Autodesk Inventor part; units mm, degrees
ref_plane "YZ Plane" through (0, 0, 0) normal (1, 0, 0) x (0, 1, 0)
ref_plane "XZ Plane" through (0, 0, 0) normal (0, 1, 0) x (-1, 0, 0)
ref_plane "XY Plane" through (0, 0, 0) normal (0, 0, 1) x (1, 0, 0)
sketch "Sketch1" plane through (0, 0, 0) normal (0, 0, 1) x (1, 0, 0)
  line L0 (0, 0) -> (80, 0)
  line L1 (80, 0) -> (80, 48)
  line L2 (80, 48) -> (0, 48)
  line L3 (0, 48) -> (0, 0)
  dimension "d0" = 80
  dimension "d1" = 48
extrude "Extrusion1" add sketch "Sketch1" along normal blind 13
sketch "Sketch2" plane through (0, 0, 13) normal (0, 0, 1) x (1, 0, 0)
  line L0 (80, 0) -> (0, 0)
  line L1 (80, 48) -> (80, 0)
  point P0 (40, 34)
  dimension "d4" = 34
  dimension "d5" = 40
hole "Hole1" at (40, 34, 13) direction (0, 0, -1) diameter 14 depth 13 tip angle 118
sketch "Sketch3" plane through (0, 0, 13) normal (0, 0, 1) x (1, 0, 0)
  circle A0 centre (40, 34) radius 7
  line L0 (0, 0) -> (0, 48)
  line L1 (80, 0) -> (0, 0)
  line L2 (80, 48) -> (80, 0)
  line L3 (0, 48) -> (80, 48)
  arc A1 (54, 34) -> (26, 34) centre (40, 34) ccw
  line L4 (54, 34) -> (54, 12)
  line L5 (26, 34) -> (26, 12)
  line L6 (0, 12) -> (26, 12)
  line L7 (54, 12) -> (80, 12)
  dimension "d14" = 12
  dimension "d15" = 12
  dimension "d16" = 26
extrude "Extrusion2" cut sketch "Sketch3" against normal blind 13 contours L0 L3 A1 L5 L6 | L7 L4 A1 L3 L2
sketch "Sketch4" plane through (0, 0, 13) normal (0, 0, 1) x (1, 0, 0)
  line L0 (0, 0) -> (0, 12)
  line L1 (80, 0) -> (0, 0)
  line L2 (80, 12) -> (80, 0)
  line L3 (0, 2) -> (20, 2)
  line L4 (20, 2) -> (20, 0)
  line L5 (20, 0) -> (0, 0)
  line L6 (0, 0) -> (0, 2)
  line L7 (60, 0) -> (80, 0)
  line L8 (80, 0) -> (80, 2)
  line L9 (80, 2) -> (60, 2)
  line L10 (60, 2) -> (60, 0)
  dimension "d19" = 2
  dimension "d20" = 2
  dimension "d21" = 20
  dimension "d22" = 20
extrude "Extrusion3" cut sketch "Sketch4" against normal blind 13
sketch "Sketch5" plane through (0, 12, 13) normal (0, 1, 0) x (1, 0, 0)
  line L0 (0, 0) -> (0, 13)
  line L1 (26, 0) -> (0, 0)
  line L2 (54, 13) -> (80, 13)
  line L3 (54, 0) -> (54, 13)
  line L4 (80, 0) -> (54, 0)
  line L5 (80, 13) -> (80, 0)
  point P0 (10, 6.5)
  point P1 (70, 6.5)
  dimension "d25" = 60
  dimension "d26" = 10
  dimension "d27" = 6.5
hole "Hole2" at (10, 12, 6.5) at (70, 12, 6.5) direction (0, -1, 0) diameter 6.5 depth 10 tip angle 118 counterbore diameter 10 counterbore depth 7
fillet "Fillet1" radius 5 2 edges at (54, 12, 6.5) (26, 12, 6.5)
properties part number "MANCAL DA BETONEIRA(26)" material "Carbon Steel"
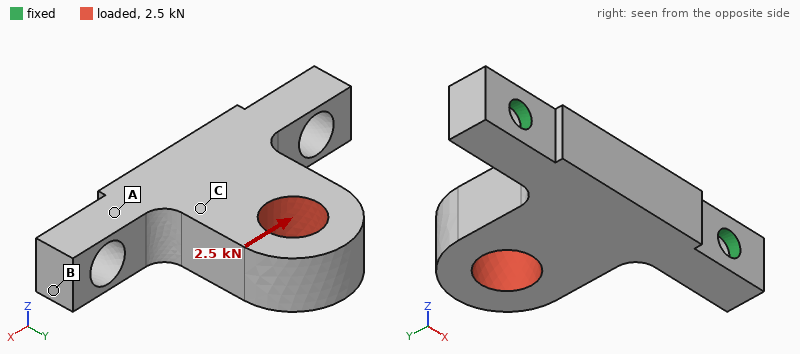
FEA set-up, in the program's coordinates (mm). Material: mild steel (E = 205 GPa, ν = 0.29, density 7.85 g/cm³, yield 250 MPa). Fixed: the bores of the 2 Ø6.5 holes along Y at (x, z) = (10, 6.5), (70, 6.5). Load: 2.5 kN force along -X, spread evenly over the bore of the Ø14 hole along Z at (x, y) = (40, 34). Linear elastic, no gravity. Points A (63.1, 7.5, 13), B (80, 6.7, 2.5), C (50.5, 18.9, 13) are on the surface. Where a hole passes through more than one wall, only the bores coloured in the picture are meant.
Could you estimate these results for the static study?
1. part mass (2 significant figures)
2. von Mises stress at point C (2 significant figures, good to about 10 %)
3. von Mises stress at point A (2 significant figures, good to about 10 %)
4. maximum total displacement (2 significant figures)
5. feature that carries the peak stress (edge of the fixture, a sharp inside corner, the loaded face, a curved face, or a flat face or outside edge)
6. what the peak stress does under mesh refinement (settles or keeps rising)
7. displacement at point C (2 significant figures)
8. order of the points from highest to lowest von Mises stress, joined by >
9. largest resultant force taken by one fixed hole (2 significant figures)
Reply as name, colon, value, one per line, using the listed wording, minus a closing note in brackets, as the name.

part mass: 160 g
von Mises stress at point C: 19 MPa
von Mises stress at point A: 33 MPa
maximum total displacement: 20 µm
feature that carries the peak stress: edge of the fixture
what the peak stress does under mesh refinement: keeps rising
displacement at point C: 5.3 µm
order of the points from highest to lowest von Mises stress, joined by >: A > C > B
largest resultant force taken by one fixed hole: 1.9 kN
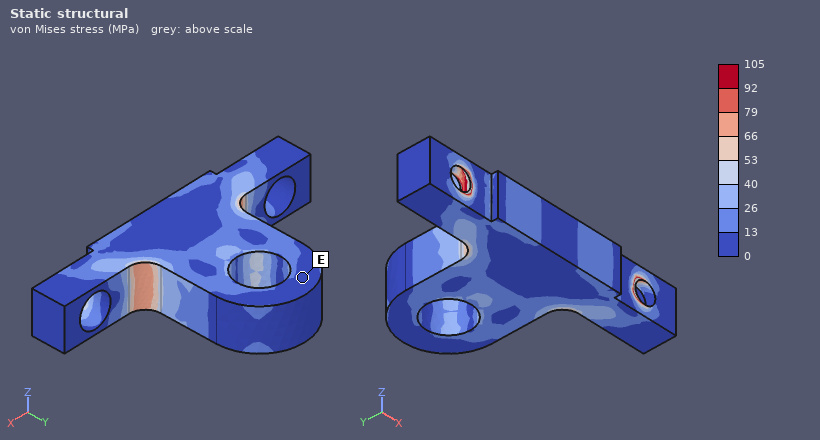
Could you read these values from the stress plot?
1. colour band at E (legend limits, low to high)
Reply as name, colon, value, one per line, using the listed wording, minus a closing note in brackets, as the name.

colour band at E: 0 to 13 MPa
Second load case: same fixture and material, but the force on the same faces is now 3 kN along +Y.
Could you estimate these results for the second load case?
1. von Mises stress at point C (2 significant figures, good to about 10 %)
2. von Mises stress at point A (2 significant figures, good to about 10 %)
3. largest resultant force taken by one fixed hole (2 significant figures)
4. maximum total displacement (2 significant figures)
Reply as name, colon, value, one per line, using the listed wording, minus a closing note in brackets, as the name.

von Mises stress at point C: 17 MPa
von Mises stress at point A: 32 MPa
largest resultant force taken by one fixed hole: 2.0 kN
maximum total displacement: 9.9 µm
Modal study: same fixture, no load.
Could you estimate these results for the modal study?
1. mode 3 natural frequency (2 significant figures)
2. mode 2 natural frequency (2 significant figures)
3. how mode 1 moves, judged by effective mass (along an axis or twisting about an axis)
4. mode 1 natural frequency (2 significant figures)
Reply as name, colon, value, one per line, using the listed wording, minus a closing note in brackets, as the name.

mode 3 natural frequency: 8800 Hz
mode 2 natural frequency: 8500 Hz
how mode 1 moves, judged by effective mass: along Z
mode 1 natural frequency: 2400 Hz
